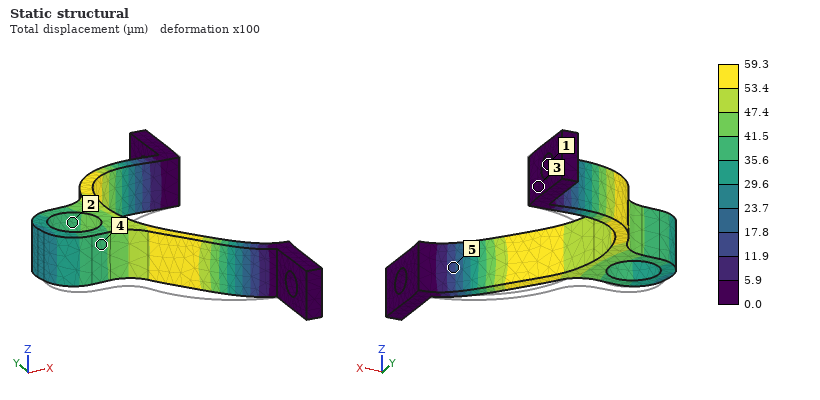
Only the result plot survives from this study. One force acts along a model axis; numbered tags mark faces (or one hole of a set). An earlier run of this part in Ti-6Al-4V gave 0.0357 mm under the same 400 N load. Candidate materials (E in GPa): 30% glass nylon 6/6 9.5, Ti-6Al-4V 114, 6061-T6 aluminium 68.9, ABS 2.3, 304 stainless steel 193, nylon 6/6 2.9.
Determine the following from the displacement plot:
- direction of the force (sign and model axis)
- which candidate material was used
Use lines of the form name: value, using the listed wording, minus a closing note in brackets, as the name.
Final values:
direction of the force: +Y
which candidate material was used: 6061-T6 aluminium
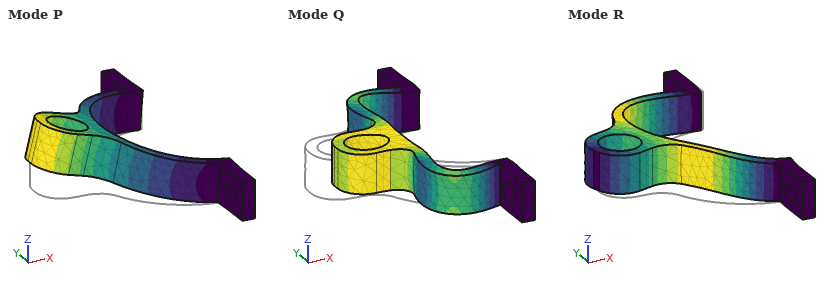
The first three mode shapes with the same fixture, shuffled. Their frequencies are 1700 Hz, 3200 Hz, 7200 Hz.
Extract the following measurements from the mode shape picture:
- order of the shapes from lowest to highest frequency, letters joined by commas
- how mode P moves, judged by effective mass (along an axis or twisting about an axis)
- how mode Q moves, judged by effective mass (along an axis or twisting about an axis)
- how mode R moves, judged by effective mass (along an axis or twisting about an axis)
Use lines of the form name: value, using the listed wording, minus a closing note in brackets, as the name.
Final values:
order of the shapes from lowest to highest frequency, letters joined by commas: P, R, Q
how mode P moves, judged by effective mass: along Z
how mode Q moves, judged by effective mass: along X
how mode R moves, judged by effective mass: along Y
